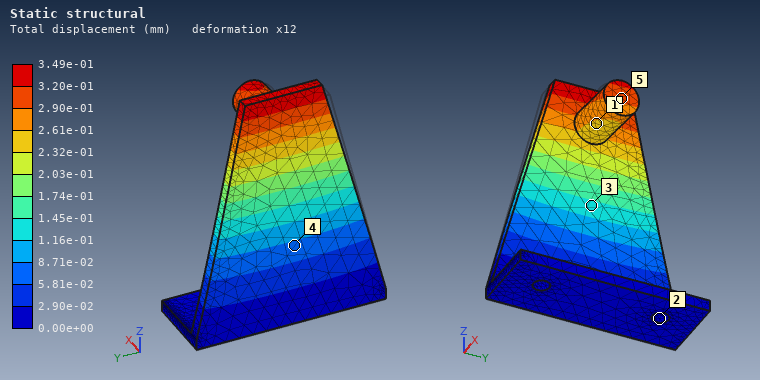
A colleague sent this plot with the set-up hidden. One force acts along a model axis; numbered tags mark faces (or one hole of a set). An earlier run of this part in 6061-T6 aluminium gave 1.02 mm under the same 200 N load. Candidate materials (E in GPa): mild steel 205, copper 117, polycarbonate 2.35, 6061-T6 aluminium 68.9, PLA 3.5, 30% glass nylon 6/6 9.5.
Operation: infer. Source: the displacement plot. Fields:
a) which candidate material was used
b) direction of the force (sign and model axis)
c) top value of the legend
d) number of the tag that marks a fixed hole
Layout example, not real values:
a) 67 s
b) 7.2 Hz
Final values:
a) mild steel
b) +X
c) 3.49e-01 mm
d) 2
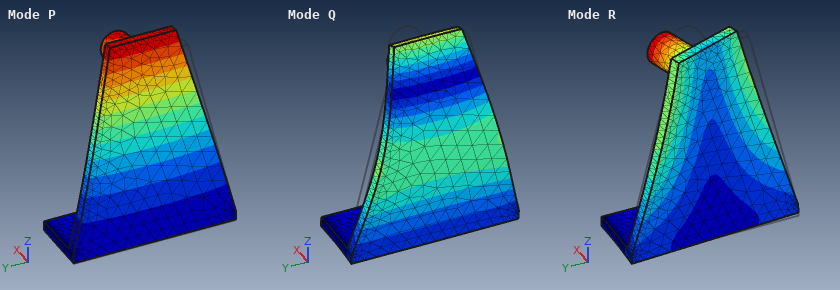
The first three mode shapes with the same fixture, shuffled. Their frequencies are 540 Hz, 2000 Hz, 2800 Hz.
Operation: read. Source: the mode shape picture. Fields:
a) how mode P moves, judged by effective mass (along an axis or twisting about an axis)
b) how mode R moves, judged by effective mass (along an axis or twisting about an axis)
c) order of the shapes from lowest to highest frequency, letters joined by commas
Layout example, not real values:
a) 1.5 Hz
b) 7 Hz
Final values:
a) along X
b) along Y
c) P, R, Q
